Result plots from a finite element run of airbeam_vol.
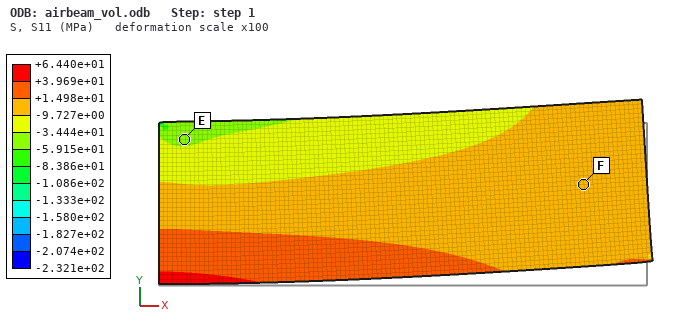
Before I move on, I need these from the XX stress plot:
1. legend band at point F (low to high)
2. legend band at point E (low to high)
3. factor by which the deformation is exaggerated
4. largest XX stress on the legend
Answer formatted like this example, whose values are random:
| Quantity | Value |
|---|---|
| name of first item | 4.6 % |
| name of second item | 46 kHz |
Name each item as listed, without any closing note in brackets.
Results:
| Quantity | Value |
|---|---|
| legend band at point F | -9.727e+00 to +1.498e+01 MPa |
| legend band at point E | -5.915e+01 to -3.444e+01 MPa |
| factor by which the deformation is exaggerated | 100 |
| largest XX stress on the legend | +6.440e+01 MPa |
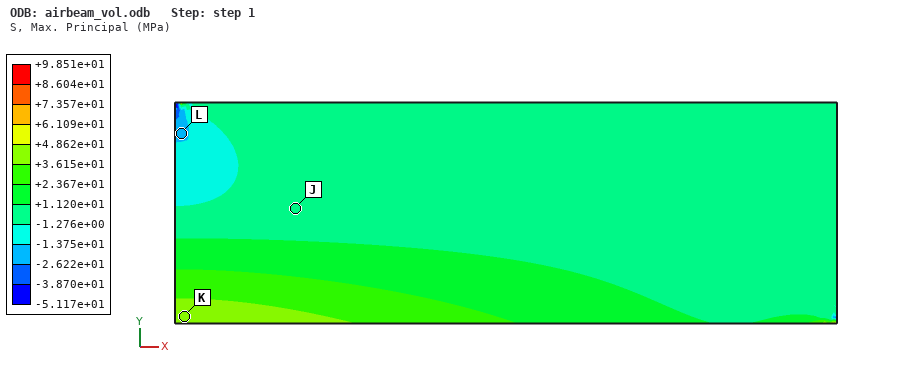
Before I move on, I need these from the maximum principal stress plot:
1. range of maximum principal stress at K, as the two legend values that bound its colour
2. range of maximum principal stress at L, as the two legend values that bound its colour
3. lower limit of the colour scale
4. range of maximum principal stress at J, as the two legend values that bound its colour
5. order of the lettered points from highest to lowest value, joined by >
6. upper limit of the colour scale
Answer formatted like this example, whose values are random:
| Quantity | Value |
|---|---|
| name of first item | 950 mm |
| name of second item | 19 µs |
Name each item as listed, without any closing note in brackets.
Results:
| Quantity | Value |
|---|---|
| range of maximum principal stress at K, as the two legend values that bound its colour | +3.615e+01 to +4.862e+01 MPa |
| range of maximum principal stress at L, as the two legend values that bound its colour | -2.622e+01 to -1.375e+01 MPa |
| lower limit of the colour scale | -5.117e+01 MPa |
| range of maximum principal stress at J, as the two legend values that bound its colour | -1.276e+00 to +1.120e+01 MPa |
| order of the lettered points from highest to lowest value, joined by > | K > J > L |
| upper limit of the colour scale | +9.851e+01 MPa |
